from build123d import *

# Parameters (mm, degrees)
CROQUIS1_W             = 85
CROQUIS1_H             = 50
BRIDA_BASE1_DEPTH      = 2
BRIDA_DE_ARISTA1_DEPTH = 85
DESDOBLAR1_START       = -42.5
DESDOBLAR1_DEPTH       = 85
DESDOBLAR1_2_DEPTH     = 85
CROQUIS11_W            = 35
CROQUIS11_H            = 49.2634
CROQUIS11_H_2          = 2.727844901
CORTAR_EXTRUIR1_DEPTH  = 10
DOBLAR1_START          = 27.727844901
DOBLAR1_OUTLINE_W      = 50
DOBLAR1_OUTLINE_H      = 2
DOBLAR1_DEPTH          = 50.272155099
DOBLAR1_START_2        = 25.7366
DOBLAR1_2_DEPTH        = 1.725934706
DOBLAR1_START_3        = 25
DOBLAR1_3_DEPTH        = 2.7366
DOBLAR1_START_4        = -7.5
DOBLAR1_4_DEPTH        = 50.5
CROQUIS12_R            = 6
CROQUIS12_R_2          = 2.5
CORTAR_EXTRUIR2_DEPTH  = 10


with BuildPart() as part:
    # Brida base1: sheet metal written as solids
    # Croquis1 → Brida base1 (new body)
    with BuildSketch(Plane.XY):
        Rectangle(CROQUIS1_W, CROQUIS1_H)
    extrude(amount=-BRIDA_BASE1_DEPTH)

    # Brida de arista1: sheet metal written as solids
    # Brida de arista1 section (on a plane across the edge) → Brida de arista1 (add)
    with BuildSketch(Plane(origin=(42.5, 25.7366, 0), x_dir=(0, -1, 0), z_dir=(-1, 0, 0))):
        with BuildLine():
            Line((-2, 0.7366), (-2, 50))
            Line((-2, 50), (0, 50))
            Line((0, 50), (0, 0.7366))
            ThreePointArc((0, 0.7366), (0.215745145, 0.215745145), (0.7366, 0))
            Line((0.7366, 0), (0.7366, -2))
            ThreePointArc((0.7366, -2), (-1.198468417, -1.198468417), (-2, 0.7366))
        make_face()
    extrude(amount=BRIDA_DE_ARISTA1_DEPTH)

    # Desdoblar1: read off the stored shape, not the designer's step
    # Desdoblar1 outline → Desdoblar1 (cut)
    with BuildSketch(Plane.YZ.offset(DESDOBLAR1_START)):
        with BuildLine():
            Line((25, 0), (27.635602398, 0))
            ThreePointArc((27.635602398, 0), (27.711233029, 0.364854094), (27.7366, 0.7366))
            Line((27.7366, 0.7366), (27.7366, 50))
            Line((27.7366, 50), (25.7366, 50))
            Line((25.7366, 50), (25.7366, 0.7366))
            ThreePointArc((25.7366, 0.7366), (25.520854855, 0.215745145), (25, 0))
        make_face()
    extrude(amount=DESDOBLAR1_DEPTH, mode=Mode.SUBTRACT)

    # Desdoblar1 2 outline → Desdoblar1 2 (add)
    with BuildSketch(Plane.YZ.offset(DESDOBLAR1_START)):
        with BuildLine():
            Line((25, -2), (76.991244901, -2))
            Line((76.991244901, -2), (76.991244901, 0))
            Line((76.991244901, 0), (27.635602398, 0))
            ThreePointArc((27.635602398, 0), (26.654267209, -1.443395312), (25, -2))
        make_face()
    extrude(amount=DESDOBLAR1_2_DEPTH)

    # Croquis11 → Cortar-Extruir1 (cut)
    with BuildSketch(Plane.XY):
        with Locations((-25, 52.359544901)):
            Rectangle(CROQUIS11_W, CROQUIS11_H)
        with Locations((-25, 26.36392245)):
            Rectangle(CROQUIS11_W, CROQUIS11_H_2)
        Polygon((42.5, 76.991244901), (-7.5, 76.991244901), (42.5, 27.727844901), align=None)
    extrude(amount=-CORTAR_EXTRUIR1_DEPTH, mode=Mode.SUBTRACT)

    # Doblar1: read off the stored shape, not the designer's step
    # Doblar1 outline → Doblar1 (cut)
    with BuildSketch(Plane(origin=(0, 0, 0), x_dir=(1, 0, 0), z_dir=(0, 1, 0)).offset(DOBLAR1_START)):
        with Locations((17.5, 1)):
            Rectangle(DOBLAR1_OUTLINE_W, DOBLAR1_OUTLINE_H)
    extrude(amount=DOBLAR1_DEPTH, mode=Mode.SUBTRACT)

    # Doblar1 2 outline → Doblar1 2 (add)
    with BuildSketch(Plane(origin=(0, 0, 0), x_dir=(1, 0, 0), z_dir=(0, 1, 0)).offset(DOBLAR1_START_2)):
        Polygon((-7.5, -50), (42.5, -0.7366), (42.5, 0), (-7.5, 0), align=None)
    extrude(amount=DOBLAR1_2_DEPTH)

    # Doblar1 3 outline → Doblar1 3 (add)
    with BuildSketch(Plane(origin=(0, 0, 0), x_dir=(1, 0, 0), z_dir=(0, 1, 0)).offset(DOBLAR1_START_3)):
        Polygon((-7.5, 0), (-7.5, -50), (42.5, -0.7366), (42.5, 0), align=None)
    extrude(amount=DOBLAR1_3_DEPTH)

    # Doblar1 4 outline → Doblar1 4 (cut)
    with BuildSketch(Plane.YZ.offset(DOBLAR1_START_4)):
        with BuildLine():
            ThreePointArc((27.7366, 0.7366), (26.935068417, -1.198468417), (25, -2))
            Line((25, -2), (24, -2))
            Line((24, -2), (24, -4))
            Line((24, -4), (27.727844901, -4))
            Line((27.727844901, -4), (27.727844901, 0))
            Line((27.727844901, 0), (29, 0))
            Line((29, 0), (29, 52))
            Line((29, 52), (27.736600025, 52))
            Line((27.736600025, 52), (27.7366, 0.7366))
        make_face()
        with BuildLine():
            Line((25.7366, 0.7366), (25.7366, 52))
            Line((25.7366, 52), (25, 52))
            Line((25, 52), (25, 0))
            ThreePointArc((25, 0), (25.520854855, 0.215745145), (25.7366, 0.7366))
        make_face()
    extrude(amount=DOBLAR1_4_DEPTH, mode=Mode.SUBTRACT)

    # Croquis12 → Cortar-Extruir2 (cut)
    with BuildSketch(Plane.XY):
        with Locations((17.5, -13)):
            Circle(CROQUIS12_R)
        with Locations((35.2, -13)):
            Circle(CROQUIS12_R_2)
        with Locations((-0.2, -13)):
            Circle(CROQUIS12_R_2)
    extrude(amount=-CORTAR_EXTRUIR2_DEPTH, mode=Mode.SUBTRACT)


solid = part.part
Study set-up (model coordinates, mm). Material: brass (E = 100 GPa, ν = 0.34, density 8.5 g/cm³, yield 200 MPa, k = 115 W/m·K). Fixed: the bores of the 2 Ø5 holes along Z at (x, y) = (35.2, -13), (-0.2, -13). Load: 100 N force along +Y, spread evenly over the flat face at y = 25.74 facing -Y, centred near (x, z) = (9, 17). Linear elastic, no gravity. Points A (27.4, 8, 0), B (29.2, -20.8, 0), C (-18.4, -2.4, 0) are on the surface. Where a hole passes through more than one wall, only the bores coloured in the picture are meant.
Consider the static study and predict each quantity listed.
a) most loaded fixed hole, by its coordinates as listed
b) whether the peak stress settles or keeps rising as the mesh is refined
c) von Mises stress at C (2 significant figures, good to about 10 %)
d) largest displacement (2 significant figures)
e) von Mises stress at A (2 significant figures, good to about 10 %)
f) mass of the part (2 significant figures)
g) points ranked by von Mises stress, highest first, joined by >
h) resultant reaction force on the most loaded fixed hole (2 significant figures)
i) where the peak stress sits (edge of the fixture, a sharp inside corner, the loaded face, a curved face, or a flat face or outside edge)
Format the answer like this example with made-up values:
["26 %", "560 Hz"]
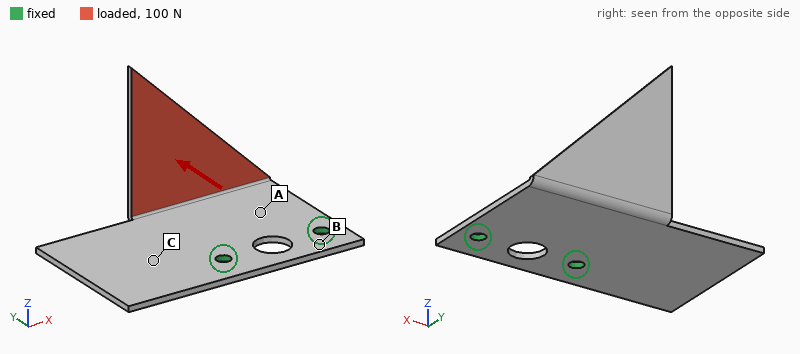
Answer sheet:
["(-0.2, -13)", "keeps rising", "24 MPa", "1.3 mm", "38 MPa", "93 g", "A > C > B", "74 N", "a sharp inside corner"]
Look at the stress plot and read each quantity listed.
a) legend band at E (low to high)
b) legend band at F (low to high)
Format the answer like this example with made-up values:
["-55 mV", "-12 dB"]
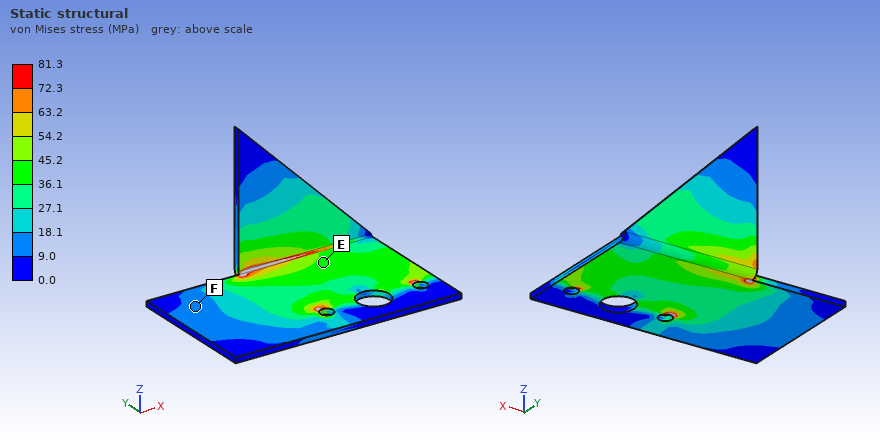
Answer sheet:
["36.1 to 45.2 MPa", "9.0 to 18.1 MPa"]
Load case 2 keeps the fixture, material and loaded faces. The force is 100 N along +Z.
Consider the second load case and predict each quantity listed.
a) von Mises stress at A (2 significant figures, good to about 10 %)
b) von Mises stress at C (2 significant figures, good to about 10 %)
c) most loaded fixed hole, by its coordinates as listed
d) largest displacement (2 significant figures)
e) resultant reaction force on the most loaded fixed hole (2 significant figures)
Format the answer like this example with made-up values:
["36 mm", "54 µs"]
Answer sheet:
["35 MPa", "37 MPa", "(-0.2, -13)", "0.95 mm", "69 N"]
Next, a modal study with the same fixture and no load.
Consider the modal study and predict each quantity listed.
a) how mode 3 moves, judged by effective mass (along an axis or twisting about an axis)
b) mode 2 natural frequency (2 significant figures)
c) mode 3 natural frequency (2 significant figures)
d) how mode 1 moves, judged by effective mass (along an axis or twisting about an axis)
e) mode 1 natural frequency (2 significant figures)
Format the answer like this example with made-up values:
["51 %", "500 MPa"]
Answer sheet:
["along Z", "500 Hz", "740 Hz", "along Z", "320 Hz"]
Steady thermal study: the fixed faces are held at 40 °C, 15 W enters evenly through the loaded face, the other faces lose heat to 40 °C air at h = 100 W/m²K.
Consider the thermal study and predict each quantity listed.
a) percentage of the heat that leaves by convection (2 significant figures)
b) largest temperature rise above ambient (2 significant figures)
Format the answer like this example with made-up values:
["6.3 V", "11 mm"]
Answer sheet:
["71 %", "43 K"]
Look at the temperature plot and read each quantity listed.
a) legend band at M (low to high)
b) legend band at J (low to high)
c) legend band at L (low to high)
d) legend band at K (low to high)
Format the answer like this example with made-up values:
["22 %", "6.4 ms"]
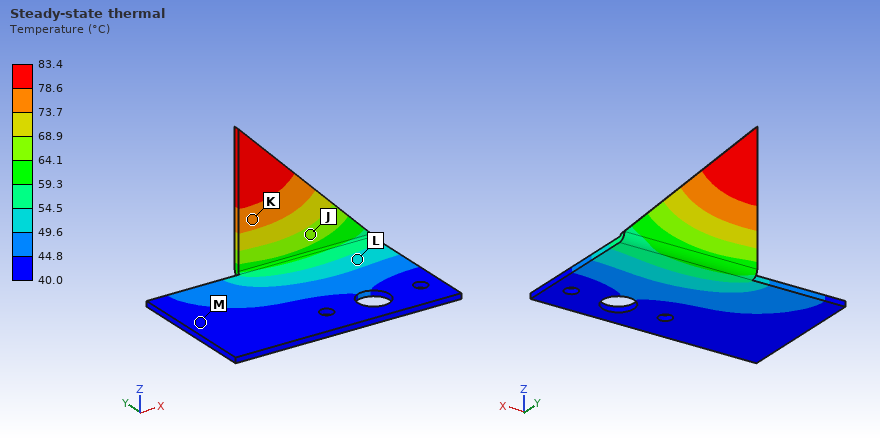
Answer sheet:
["40.0 to 44.8 °C", "64.1 to 68.9 °C", "49.6 to 54.5 °C", "73.7 to 78.6 °C"]
